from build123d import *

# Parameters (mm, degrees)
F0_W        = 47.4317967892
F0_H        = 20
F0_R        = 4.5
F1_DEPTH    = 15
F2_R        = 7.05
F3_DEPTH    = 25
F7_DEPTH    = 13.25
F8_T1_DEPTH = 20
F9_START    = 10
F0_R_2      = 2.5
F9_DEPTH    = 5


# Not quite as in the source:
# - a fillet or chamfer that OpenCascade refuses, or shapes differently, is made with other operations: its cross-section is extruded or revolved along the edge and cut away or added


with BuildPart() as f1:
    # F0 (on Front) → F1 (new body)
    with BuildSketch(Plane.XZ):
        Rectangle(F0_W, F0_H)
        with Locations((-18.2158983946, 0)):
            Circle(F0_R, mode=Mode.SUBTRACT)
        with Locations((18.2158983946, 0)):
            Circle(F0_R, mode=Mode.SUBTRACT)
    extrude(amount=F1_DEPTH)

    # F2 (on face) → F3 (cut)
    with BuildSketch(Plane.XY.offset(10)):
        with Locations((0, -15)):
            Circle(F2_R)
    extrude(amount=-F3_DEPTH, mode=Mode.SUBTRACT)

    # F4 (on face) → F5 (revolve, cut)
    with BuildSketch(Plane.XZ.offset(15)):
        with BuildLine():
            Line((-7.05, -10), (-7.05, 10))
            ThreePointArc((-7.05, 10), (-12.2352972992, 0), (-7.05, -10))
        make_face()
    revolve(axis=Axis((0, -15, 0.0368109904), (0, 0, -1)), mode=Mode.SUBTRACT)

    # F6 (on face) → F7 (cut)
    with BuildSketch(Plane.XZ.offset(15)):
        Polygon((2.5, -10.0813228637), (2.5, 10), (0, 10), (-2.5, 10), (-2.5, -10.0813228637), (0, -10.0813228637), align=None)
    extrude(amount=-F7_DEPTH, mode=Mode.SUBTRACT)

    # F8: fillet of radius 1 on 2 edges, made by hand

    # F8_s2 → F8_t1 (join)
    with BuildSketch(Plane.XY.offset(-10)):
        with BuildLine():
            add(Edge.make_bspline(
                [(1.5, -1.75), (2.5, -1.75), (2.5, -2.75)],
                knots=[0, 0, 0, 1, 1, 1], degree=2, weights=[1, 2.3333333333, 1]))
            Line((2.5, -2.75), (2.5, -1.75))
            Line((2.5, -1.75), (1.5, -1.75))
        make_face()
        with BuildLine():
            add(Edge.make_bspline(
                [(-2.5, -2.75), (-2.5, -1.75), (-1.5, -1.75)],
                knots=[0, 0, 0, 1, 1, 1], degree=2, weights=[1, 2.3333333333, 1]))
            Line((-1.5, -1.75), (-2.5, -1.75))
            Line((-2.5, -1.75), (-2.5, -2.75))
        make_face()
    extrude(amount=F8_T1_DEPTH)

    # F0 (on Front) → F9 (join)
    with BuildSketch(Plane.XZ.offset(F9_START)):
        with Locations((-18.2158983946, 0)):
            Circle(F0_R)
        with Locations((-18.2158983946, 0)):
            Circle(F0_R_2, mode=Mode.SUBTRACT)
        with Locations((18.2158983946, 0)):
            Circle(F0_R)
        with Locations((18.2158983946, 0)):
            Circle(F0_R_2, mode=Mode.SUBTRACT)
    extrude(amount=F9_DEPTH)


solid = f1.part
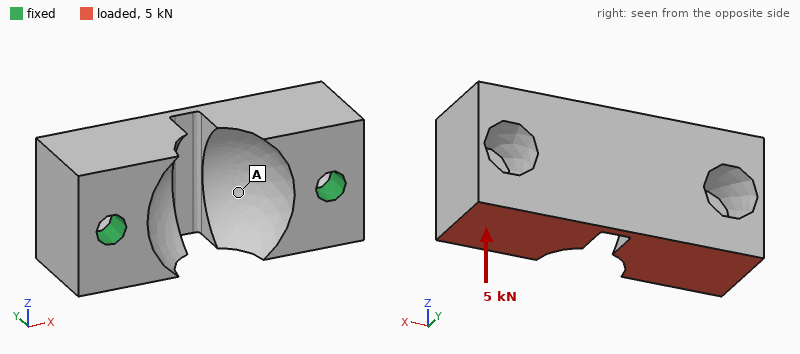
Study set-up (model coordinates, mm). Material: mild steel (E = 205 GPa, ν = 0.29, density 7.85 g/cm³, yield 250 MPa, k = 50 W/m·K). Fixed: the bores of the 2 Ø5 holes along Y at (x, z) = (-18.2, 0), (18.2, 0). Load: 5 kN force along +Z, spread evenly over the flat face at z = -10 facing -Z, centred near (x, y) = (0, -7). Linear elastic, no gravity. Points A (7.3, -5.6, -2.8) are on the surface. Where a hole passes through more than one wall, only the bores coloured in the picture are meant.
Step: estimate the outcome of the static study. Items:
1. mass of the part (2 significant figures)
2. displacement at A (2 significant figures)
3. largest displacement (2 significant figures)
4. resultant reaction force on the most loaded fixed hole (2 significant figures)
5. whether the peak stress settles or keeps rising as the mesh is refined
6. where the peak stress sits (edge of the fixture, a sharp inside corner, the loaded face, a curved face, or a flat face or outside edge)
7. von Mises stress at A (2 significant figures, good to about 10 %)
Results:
69 g
8.2 µm
15 µm
2.5 kN
keeps rising
edge of the fixture
23 MPa
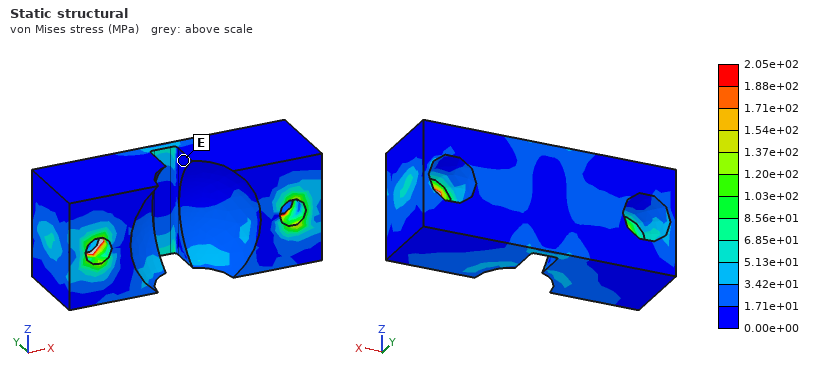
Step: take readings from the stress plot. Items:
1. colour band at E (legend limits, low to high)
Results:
0.00e+00 to 1.71e+01 MPa
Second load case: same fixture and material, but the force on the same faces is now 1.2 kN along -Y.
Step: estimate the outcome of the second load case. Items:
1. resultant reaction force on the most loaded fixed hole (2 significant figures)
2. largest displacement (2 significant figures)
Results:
620 N
5.4 µm
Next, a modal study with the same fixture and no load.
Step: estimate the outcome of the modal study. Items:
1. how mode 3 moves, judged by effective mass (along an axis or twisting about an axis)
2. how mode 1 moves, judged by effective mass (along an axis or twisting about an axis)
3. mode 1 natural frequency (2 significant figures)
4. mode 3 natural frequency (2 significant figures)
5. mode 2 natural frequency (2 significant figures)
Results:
along X
along Z
13 kHz
19 kHz
18 kHz
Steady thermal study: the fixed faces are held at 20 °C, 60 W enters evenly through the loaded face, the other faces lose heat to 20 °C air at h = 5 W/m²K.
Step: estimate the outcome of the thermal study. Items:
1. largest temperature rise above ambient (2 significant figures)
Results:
63 K
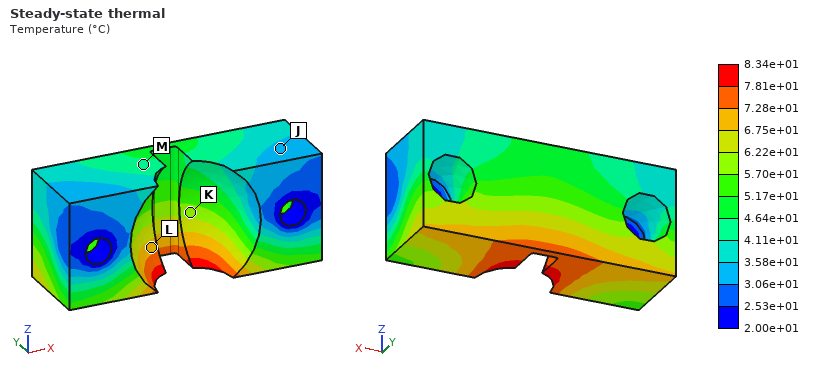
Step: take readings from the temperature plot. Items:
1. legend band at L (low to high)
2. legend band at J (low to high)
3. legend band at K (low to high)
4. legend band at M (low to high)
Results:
6.75e+01 to 7.28e+01 °C
3.06e+01 to 3.58e+01 °C
5.70e+01 to 6.22e+01 °C
4.11e+01 to 4.64e+01 °C
